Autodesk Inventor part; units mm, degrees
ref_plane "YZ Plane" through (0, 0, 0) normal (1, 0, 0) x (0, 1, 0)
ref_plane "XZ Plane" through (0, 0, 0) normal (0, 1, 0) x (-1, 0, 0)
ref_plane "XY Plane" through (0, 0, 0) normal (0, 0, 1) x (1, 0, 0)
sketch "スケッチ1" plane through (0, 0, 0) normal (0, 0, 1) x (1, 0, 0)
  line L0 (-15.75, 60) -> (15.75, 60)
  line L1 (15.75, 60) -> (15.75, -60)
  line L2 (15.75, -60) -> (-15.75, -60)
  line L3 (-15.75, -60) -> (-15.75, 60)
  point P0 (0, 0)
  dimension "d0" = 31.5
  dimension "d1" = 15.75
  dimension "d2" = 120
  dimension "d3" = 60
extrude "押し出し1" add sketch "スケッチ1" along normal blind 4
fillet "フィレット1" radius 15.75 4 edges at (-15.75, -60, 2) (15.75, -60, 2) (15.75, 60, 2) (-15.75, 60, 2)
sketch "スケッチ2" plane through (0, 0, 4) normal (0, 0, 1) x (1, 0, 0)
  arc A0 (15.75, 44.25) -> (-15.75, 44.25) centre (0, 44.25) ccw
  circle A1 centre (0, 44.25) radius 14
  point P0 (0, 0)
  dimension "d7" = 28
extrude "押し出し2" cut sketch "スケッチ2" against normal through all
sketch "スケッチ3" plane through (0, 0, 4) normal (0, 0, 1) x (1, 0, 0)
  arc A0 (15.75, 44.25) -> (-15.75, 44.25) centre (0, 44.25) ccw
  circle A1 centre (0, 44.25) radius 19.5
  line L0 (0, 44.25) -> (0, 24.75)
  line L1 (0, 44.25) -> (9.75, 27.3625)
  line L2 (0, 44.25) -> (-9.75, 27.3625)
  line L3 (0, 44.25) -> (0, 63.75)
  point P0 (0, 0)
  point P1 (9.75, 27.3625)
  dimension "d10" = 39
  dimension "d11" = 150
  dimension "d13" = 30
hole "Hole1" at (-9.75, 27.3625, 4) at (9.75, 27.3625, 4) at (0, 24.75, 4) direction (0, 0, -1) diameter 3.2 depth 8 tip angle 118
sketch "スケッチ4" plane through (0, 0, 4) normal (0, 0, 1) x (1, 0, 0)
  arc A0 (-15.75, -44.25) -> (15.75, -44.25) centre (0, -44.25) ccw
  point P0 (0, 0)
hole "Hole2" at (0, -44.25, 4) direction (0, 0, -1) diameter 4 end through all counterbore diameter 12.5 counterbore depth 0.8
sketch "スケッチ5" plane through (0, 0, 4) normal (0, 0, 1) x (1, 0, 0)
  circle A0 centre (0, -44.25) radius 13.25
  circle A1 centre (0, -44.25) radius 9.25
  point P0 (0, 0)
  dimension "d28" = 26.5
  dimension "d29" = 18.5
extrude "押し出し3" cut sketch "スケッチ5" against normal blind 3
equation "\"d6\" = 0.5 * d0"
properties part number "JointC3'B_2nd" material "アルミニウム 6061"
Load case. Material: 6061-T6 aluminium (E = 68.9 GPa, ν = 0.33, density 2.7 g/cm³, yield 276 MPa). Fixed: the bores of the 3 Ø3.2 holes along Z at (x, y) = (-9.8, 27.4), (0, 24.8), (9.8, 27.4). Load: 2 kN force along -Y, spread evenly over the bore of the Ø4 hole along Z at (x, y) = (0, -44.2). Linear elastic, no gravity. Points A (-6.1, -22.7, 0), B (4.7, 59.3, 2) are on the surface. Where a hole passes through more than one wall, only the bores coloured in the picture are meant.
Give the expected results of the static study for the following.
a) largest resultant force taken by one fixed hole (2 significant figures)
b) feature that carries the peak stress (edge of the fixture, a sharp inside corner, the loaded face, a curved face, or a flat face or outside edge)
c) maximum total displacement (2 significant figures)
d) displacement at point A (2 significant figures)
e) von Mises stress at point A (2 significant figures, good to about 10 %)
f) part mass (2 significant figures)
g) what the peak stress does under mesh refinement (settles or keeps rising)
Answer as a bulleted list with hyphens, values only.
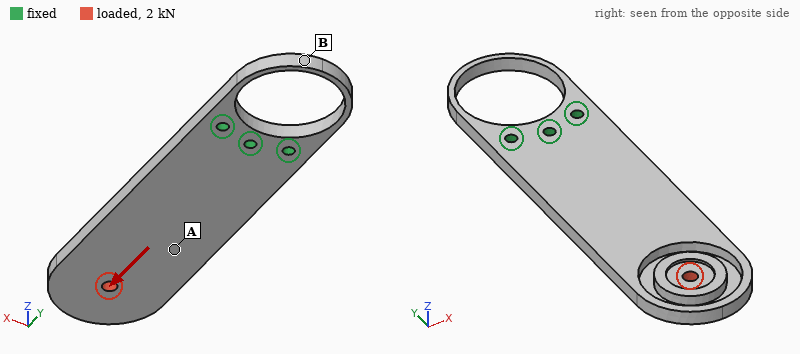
- 680 N
- a sharp inside corner
- 0.14 mm
- 0.082 mm
- 28 MPa
- 29 g
- keeps rising
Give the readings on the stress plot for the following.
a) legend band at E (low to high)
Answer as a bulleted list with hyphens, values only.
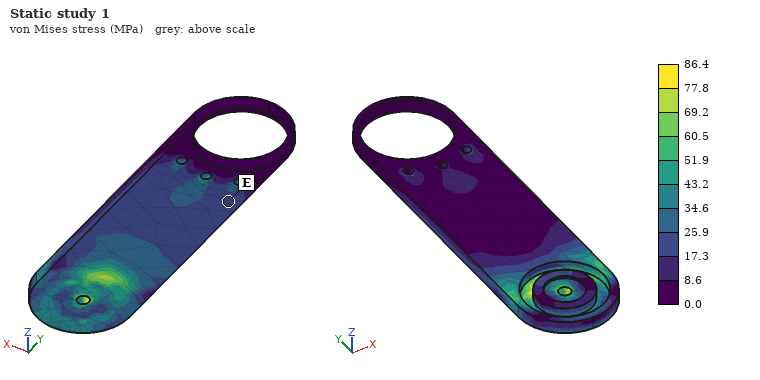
- 17.3 to 25.9 MPa
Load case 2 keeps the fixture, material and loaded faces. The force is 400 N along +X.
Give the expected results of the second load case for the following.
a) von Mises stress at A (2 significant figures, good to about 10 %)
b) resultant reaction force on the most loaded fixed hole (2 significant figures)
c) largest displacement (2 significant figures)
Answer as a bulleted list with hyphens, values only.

- 8.7 MPa
- 1.3 kN
- 0.12 mm
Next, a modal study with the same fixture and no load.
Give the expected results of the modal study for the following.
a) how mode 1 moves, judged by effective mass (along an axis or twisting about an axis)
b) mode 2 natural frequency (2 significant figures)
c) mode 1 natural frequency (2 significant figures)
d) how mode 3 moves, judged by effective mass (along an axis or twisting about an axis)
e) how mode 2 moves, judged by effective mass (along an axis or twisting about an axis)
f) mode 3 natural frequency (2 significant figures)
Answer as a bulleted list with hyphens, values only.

- along Z
- 2700 Hz
- 560 Hz
- along Z
- twisting about Y
- 2900 Hz
